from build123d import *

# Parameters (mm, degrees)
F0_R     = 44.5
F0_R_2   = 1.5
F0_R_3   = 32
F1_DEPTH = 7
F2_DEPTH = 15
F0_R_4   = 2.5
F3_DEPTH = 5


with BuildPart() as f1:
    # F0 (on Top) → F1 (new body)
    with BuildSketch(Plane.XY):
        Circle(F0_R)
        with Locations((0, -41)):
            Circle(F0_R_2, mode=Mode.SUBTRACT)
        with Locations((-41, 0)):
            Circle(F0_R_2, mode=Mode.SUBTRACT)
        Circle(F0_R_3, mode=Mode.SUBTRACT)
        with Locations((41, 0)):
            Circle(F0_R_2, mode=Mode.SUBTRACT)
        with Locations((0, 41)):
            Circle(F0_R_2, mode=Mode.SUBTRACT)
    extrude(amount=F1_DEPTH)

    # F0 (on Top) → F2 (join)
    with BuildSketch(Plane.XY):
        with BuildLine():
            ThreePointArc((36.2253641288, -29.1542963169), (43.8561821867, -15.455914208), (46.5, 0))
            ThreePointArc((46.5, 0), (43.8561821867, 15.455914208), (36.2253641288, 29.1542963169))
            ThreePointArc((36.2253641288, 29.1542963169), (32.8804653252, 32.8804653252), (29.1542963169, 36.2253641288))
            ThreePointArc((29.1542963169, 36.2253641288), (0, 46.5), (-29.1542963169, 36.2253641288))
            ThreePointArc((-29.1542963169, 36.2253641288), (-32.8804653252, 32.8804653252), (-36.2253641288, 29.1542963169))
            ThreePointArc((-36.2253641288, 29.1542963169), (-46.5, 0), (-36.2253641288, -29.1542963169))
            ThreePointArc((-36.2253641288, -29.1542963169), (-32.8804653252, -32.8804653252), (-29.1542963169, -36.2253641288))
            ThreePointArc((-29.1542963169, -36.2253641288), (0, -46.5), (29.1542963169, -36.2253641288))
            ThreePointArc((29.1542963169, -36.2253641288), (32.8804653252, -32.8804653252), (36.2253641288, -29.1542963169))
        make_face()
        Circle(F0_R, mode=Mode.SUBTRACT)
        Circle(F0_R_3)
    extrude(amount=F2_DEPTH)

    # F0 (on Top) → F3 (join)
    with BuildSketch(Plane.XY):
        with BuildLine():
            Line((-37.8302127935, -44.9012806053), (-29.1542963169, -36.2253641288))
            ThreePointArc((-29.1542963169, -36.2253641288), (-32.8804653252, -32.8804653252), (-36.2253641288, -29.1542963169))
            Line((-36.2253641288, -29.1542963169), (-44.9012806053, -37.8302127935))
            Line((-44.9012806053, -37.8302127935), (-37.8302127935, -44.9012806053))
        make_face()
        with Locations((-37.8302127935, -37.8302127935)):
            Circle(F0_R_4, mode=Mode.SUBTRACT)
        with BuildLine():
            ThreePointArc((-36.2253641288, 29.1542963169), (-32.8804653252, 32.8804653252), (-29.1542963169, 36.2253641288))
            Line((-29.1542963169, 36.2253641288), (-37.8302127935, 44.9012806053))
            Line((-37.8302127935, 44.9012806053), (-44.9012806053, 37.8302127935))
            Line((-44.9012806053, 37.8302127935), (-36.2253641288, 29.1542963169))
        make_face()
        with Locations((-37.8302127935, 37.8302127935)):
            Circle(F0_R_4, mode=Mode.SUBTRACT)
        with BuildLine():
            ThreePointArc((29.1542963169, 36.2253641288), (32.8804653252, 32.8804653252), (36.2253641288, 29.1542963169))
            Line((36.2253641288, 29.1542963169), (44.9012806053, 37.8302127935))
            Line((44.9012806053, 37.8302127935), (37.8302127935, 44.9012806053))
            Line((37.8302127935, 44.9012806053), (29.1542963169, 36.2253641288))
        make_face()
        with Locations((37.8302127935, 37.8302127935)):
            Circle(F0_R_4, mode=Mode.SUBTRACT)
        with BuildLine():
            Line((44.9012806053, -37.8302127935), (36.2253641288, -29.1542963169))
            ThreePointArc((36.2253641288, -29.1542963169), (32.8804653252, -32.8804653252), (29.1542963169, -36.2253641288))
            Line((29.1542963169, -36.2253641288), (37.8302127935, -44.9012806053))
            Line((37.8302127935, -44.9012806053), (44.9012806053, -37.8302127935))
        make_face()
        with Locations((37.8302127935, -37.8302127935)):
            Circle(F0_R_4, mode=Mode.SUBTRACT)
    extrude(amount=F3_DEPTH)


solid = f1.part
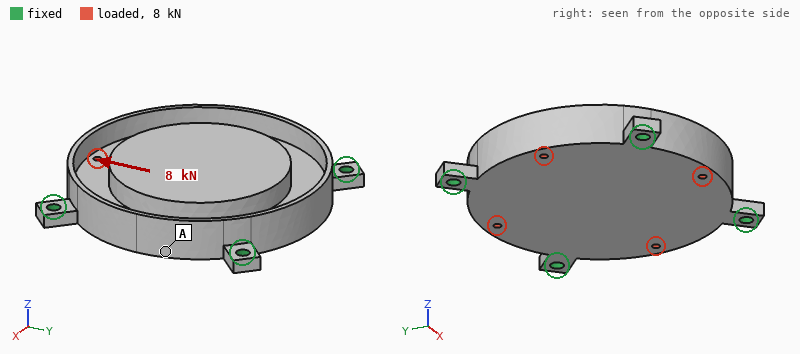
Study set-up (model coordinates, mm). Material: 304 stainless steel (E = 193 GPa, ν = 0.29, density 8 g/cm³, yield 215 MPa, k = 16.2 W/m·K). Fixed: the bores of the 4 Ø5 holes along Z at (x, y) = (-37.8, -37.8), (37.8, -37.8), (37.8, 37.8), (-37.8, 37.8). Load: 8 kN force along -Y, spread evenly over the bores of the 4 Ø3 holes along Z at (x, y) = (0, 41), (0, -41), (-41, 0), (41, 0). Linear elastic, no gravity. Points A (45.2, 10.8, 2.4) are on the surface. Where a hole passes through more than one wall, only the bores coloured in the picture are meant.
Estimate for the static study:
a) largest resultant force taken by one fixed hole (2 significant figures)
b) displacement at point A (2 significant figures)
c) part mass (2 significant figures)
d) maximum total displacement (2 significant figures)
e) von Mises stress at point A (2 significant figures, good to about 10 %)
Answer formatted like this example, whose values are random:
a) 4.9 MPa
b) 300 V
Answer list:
a) 2.1 kN
b) 4.9 µm
c) 640 g
d) 7.0 µm
e) 8.5 MPa
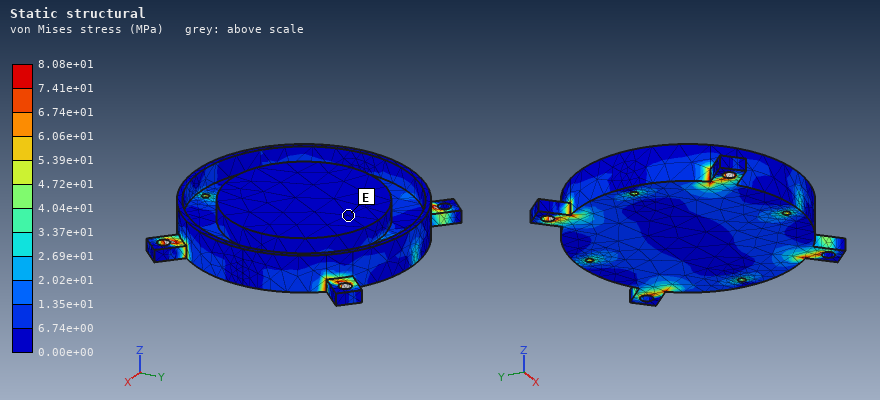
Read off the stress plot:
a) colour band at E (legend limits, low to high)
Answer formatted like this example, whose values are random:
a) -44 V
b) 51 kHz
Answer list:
a) 0.00e+00 to 6.74e+00 MPa
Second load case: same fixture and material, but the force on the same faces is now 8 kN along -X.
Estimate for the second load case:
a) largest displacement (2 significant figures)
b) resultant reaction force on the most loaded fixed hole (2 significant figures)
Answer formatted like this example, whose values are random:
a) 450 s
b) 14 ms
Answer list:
a) 7.0 µm
b) 2.1 kN
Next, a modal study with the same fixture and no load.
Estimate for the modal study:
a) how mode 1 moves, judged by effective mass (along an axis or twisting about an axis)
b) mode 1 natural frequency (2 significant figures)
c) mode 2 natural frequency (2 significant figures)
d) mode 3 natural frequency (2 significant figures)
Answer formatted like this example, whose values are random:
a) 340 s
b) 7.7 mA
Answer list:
a) along Z
b) 3500 Hz
c) 5300 Hz
d) 5300 Hz
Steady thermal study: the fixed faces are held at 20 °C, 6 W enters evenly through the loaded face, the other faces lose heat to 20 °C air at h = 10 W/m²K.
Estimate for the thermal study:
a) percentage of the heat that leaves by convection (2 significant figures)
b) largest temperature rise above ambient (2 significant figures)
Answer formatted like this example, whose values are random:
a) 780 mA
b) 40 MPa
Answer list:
a) 42 %
b) 18 K
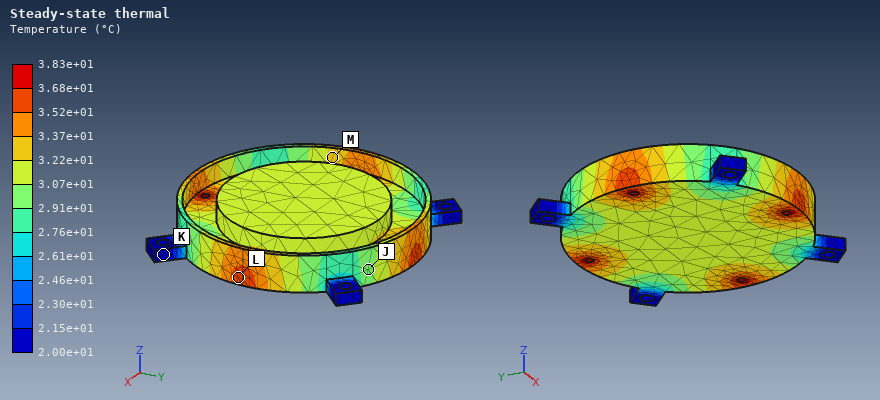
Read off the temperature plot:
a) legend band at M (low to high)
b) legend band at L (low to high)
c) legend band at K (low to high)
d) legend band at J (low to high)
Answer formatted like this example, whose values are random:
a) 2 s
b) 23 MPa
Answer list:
a) 3.22e+01 to 3.37e+01 °C
b) 3.52e+01 to 3.68e+01 °C
c) 2.00e+01 to 2.15e+01 °C
d) 2.91e+01 to 3.07e+01 °C
